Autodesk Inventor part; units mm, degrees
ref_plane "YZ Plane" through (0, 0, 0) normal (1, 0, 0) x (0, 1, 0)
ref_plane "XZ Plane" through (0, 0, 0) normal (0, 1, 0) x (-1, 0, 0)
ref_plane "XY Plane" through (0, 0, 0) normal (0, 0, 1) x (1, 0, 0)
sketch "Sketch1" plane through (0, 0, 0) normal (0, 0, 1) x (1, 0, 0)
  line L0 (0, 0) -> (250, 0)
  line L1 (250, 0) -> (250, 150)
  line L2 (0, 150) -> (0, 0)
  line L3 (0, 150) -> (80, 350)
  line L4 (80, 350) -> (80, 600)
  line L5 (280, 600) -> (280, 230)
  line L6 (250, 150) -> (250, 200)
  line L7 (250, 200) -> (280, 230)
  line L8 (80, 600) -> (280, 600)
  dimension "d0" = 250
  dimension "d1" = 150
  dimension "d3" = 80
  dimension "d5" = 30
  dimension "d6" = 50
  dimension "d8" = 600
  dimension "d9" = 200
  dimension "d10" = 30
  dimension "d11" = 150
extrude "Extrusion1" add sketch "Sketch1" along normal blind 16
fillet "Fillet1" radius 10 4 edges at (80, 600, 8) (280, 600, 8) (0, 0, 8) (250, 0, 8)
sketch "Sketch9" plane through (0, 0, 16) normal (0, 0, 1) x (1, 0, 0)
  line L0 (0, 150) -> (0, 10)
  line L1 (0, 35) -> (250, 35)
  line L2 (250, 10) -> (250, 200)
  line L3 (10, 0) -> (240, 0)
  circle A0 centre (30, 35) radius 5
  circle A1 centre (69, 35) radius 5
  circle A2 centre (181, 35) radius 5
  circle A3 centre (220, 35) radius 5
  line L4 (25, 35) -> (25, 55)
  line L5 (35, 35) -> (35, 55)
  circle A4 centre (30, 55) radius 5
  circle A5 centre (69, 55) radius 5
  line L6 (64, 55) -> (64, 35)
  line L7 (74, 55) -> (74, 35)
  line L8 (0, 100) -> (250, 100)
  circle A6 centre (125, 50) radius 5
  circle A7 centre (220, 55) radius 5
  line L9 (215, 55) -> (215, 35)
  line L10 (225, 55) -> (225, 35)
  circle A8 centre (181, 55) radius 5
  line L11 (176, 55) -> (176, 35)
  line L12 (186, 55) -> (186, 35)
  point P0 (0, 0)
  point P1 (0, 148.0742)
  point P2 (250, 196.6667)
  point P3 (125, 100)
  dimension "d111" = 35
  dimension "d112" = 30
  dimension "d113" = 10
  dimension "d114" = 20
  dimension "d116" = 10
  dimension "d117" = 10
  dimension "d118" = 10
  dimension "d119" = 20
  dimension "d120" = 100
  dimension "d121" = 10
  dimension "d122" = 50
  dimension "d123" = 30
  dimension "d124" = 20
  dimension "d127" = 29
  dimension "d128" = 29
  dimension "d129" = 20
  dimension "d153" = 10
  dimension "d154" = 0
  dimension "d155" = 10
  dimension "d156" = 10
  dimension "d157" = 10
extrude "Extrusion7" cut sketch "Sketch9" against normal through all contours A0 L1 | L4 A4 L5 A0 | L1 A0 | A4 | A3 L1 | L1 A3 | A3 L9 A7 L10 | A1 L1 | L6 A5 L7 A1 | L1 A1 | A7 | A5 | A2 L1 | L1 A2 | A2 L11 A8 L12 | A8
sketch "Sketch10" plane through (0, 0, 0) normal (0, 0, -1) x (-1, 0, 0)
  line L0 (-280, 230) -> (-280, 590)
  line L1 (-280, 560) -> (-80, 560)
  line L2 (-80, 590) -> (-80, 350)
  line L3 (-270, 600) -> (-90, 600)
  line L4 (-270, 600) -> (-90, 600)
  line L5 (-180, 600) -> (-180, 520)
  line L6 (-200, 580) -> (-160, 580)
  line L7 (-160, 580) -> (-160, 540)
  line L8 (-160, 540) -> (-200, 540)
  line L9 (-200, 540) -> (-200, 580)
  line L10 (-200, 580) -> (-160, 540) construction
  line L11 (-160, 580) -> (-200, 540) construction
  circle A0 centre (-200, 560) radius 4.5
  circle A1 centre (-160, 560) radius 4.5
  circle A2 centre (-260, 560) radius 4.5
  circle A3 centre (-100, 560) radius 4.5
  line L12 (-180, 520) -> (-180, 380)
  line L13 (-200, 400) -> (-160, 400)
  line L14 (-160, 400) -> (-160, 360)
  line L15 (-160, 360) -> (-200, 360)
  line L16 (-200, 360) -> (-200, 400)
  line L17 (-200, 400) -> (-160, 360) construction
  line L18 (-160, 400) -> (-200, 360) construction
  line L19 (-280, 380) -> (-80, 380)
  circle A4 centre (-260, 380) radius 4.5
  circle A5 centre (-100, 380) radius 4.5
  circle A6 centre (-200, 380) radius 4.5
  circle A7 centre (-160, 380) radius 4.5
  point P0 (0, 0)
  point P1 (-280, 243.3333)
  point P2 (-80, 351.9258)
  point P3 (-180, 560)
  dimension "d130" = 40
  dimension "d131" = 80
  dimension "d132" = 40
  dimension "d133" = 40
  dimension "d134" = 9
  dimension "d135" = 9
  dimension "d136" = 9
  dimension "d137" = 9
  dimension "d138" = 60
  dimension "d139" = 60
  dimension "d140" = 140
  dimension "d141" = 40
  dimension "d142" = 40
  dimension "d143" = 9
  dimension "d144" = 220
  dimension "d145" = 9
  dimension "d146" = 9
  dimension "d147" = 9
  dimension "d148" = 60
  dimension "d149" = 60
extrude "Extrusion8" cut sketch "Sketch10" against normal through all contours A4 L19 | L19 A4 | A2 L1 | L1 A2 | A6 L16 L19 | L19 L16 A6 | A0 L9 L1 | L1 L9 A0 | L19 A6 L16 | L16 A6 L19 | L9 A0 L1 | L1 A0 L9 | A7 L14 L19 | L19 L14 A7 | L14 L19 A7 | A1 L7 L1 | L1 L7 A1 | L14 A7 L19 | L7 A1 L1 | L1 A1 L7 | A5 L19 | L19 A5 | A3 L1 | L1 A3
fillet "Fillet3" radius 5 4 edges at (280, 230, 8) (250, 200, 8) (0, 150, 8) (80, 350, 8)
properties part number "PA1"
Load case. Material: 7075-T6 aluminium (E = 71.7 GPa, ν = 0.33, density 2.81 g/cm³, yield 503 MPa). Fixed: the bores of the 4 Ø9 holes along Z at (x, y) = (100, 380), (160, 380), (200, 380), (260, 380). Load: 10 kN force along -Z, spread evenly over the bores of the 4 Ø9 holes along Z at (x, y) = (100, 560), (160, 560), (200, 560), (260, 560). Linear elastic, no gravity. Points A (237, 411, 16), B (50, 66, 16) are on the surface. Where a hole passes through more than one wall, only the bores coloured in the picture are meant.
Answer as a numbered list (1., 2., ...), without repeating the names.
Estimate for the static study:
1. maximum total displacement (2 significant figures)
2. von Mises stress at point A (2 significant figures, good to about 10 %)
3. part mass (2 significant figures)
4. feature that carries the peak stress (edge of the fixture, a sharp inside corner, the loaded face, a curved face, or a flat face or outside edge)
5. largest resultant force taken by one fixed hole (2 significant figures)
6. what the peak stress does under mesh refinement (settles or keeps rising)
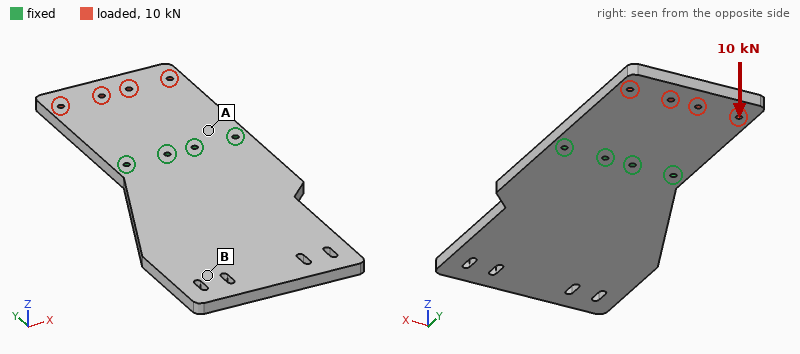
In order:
1. 5.3 mm
2. 150 MPa
3. 5.9 kg
4. edge of the fixture
5. 4.7 kN
6. keeps rising
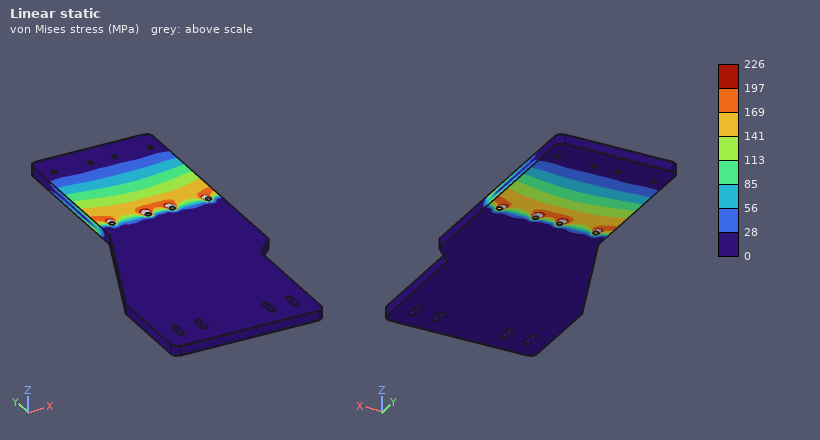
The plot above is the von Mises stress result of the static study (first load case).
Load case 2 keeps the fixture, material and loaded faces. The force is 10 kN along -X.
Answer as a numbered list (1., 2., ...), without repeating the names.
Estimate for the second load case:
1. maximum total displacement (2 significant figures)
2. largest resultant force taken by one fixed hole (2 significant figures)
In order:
1. 68 µm
2. 11 kN
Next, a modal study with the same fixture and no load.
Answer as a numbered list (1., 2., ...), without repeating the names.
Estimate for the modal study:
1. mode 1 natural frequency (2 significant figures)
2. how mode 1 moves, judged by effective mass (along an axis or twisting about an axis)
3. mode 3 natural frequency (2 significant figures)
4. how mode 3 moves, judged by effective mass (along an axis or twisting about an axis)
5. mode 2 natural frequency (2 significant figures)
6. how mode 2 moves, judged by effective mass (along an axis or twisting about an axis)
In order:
1. 84 Hz
2. along Z
3. 280 Hz
4. twisting about Y
5. 270 Hz
6. along Z
